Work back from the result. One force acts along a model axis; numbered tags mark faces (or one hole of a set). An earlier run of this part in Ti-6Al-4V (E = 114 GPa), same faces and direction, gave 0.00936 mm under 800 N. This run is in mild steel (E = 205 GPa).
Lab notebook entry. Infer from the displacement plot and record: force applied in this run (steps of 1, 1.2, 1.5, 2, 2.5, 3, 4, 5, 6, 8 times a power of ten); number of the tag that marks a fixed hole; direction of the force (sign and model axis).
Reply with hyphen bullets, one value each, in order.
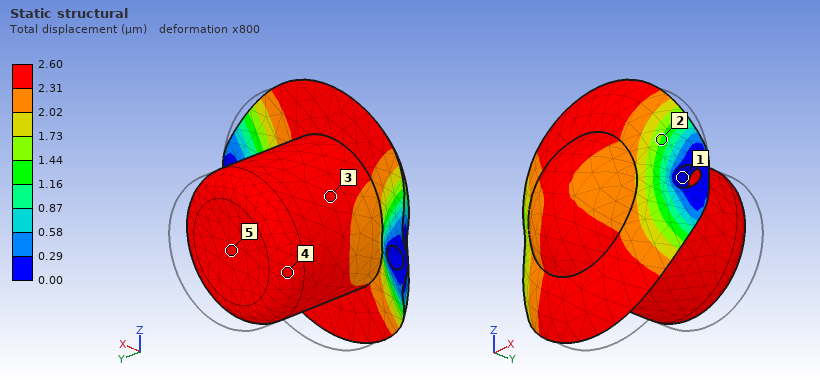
- 400 N
- 1
- -Y
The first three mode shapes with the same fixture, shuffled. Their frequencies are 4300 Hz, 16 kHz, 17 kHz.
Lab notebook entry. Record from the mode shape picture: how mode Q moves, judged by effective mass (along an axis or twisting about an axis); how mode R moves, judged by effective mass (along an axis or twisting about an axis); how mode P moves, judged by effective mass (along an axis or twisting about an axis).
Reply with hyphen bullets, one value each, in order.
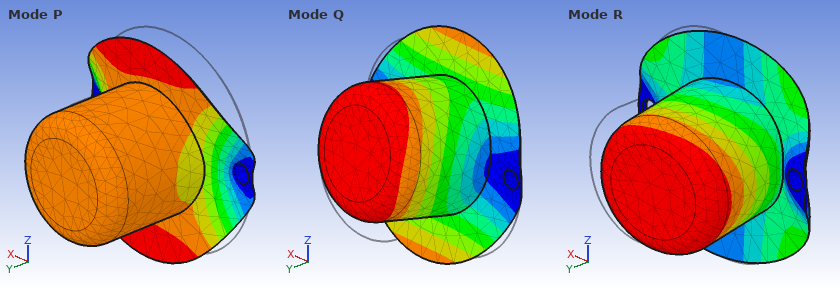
- along Z
- along X
- along Y
